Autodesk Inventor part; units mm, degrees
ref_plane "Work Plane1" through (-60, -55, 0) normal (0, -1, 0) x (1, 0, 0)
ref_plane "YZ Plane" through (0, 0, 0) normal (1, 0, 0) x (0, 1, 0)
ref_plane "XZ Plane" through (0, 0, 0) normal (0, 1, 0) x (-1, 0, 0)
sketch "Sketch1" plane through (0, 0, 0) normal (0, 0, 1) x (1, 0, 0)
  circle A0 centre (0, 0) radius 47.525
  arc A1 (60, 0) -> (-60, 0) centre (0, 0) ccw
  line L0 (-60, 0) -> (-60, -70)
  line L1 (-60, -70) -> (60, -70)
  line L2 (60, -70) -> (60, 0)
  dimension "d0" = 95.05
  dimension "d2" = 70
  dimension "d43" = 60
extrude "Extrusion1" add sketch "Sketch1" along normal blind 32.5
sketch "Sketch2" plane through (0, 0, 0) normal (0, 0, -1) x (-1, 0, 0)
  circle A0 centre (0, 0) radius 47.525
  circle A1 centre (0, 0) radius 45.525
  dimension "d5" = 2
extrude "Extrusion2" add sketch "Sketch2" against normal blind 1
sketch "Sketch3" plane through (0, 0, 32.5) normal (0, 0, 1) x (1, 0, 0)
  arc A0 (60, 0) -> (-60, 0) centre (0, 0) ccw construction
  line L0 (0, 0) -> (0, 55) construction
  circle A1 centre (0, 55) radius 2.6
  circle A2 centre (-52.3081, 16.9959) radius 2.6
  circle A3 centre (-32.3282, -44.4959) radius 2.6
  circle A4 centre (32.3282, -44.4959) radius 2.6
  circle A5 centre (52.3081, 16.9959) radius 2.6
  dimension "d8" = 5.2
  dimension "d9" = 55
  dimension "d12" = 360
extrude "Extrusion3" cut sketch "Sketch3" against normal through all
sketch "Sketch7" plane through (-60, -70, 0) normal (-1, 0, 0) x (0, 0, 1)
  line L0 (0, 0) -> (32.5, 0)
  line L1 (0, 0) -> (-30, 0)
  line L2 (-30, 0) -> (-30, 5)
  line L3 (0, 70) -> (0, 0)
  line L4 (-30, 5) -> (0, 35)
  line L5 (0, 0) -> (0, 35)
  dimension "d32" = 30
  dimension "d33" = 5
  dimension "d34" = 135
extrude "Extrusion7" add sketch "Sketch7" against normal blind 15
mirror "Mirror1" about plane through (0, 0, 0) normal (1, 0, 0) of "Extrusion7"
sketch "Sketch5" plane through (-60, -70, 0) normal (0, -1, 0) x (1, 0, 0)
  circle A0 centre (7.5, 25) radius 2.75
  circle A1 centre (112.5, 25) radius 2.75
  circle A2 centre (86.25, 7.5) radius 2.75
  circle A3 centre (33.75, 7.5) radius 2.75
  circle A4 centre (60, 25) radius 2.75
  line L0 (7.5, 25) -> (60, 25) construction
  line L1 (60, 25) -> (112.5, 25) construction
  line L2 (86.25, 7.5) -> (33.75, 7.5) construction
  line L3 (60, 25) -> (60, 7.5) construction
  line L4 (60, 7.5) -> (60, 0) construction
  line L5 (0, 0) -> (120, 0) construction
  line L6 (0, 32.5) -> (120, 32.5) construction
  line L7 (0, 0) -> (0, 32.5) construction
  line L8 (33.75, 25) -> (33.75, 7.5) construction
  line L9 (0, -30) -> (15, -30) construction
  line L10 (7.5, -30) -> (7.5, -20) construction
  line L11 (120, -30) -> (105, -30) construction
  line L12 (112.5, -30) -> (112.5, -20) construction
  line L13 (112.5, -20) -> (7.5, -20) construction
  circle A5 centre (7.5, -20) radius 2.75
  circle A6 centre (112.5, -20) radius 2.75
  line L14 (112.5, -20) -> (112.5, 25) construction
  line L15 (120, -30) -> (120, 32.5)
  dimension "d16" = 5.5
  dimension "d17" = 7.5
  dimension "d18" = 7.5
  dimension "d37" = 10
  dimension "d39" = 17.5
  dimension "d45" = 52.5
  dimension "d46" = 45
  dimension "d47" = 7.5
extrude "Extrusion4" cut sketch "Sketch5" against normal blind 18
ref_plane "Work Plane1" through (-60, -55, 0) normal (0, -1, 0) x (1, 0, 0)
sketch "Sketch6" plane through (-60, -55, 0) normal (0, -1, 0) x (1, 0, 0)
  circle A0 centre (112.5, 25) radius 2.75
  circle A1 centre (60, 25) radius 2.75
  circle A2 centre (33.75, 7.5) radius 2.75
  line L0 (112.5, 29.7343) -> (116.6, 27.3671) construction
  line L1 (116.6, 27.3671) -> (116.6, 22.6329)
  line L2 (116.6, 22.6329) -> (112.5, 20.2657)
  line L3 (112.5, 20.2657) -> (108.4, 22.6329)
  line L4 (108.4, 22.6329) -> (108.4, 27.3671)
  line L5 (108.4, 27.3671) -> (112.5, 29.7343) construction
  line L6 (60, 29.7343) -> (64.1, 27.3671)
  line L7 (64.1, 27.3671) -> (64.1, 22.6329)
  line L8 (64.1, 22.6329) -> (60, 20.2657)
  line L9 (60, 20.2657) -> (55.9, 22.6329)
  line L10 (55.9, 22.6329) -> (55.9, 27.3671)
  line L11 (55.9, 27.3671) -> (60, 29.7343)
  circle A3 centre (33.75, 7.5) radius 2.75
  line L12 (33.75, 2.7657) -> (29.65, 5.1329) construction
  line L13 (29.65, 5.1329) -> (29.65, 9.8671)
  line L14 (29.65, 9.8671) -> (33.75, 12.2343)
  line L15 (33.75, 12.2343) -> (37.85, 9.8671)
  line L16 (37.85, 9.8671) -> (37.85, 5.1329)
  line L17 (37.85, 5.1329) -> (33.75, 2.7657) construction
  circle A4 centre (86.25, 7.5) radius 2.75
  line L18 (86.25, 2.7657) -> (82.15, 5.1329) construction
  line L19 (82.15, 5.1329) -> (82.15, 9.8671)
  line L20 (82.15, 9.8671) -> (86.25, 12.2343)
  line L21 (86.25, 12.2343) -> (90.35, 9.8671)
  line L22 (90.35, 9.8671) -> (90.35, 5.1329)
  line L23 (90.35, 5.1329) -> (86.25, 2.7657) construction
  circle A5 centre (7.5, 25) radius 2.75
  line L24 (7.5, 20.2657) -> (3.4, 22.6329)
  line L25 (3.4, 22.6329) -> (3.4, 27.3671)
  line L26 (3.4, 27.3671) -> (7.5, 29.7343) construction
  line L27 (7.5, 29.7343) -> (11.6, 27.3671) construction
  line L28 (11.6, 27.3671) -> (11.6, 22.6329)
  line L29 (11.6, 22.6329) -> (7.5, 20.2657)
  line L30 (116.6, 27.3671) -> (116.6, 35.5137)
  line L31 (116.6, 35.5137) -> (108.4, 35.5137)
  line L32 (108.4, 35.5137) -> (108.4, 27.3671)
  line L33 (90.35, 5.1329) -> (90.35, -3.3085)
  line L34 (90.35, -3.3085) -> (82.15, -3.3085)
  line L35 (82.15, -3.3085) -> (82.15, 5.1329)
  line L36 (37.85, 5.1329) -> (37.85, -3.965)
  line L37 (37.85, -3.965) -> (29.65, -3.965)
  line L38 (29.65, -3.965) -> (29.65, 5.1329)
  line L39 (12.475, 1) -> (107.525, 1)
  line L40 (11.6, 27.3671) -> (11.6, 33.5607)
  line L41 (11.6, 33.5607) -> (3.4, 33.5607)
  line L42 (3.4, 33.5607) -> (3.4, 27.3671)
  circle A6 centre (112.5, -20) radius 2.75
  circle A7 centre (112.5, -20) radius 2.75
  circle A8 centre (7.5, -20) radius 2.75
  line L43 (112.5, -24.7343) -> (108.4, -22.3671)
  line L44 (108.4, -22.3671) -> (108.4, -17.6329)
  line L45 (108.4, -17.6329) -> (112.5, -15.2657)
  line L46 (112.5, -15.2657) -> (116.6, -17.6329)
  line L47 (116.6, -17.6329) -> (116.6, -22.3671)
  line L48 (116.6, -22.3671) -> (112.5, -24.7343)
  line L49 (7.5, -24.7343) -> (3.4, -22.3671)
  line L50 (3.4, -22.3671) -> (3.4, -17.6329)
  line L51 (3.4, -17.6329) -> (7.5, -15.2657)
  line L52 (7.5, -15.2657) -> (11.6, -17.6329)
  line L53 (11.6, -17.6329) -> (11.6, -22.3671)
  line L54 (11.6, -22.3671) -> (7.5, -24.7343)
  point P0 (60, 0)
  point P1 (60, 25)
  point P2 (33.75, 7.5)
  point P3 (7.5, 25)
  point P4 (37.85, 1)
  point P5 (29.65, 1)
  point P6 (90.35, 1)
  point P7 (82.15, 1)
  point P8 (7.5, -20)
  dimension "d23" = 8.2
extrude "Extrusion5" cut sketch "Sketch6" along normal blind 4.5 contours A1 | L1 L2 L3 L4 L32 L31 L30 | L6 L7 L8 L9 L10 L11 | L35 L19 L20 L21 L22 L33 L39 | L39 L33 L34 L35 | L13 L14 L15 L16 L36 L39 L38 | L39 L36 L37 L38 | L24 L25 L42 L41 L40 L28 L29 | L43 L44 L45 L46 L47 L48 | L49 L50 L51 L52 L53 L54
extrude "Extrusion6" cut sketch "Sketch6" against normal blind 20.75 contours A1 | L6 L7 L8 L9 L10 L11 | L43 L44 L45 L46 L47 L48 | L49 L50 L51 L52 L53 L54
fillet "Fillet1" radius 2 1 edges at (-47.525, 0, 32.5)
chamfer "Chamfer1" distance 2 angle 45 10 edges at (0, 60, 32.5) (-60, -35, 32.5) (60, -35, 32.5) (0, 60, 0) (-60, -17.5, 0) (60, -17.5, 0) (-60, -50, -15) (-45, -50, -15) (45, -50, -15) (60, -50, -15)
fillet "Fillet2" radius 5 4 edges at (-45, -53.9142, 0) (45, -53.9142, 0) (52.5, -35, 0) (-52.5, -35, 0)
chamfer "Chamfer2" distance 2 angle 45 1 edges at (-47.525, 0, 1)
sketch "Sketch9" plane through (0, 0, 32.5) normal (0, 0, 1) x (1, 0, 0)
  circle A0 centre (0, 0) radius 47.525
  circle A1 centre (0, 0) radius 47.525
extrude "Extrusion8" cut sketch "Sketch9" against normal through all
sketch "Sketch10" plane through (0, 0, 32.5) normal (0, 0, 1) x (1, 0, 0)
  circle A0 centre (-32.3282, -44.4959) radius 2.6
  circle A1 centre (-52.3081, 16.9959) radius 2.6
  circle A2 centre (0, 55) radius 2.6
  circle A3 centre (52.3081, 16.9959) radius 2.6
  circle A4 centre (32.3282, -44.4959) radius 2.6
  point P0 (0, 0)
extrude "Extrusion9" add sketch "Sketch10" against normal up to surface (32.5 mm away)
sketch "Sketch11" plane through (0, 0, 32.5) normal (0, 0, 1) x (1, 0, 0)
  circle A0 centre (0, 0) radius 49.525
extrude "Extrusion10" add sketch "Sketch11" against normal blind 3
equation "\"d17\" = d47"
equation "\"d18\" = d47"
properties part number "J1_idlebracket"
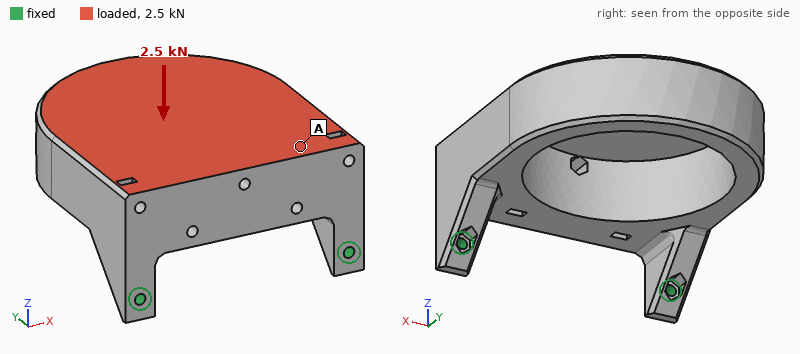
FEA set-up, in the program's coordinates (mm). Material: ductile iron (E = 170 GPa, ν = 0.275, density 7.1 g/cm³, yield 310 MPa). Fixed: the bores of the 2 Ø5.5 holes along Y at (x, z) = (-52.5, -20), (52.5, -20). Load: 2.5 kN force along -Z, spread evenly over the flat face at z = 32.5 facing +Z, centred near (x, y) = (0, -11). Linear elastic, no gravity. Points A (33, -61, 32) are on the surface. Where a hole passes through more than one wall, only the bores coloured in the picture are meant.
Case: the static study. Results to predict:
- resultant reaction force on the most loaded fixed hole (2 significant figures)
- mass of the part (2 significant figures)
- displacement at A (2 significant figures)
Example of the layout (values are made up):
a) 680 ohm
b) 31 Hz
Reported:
a) 1.3 kN
b) 1.8 kg
c) 0.085 mm
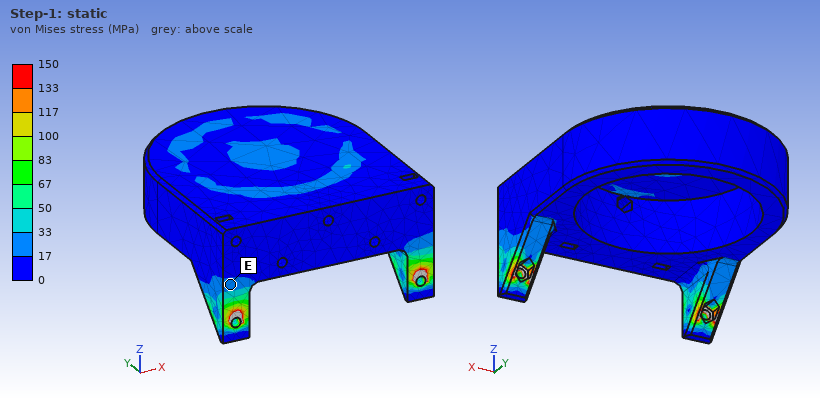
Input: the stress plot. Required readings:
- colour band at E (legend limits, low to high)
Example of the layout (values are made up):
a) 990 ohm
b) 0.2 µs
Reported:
a) 17 to 33 MPa
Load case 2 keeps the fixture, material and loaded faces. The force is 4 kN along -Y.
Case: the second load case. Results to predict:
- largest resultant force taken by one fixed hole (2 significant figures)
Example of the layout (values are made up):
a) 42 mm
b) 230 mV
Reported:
a) 2.0 kN
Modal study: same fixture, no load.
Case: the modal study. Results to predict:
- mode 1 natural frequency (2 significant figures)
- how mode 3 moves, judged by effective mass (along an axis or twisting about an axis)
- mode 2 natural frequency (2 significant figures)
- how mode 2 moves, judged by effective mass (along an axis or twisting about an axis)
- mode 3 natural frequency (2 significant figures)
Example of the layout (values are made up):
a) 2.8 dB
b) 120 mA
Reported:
a) 470 Hz
b) along Y
c) 1300 Hz
d) along X
e) 2700 Hz
